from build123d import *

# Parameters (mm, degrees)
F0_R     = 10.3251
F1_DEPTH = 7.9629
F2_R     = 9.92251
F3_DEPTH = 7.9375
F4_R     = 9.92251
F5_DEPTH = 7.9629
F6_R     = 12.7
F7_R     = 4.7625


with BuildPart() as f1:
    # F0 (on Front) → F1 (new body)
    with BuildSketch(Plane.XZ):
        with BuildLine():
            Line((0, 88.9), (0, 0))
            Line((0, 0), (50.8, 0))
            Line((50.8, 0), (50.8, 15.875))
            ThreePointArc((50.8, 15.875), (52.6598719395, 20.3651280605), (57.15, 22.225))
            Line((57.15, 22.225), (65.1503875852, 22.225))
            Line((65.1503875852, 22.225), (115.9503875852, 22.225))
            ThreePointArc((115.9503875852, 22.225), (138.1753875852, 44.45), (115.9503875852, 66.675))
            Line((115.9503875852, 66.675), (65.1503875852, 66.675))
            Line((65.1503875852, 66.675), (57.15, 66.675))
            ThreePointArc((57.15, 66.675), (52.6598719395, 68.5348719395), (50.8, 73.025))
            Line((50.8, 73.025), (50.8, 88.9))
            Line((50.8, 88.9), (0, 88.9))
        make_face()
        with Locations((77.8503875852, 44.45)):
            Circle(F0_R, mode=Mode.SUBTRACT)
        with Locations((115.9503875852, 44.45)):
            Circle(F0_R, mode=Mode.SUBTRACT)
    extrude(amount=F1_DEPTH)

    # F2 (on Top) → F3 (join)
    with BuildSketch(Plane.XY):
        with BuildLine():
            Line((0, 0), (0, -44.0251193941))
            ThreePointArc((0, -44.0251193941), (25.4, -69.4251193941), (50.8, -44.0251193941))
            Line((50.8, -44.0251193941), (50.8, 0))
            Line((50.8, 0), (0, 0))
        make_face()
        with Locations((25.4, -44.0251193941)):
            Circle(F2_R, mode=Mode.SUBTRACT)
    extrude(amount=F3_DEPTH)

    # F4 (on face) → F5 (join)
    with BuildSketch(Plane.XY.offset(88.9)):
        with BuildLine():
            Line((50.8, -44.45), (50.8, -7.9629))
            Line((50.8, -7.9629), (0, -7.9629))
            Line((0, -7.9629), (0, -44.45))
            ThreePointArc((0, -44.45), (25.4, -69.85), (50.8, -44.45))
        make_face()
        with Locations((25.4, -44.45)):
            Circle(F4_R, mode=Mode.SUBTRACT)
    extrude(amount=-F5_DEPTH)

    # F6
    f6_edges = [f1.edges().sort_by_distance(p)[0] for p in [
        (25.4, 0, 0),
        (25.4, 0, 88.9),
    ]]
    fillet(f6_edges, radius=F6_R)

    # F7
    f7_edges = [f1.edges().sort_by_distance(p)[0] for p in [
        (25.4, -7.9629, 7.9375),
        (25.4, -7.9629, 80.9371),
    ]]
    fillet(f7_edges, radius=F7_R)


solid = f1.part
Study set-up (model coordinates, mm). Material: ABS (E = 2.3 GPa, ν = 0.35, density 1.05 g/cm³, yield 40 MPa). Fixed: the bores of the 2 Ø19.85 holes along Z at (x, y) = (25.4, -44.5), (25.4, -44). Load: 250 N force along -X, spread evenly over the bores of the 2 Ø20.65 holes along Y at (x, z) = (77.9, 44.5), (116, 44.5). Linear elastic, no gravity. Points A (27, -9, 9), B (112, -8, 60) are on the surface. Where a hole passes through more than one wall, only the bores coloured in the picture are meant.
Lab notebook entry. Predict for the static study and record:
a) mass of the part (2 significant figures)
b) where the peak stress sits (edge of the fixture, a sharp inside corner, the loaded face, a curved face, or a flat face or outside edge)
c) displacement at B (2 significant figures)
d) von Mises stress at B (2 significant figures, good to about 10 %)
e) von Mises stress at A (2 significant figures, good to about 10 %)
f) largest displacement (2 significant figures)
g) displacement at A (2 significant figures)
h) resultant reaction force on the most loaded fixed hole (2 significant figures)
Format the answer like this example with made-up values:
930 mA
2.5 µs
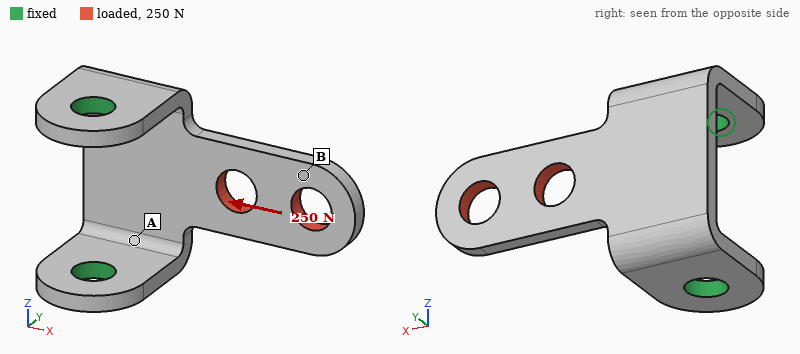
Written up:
100 g
edge of the fixture
0.12 mm
0.50 MPa
1.1 MPa
0.15 mm
0.035 mm
130 N
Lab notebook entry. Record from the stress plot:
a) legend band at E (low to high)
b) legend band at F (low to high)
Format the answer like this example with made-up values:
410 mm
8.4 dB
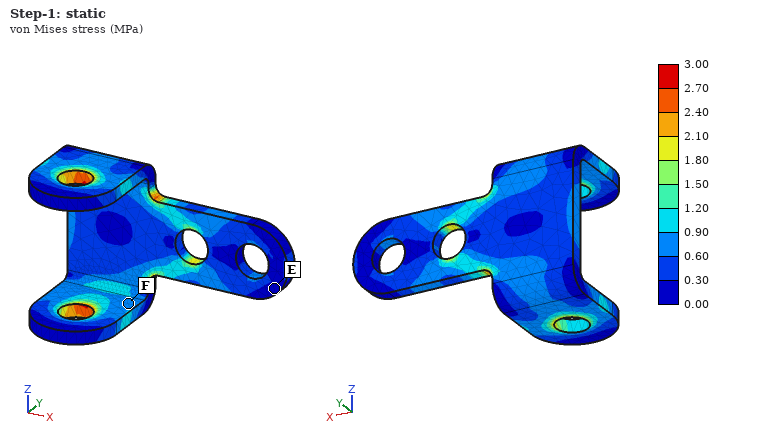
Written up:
0.00 to 0.30 MPa
0.60 to 0.90 MPa
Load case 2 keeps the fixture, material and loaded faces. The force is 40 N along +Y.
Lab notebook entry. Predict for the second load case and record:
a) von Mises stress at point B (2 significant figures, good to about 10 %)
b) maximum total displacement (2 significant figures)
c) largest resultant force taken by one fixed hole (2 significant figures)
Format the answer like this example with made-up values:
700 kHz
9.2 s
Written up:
0.44 MPa
2.0 mm
27 N
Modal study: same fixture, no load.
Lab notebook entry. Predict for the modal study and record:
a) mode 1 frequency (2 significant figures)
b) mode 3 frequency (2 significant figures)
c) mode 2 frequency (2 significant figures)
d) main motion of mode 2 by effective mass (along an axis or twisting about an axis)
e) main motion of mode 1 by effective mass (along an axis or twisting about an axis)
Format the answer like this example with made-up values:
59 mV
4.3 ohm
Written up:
190 Hz
850 Hz
670 Hz
along Z
along Y
